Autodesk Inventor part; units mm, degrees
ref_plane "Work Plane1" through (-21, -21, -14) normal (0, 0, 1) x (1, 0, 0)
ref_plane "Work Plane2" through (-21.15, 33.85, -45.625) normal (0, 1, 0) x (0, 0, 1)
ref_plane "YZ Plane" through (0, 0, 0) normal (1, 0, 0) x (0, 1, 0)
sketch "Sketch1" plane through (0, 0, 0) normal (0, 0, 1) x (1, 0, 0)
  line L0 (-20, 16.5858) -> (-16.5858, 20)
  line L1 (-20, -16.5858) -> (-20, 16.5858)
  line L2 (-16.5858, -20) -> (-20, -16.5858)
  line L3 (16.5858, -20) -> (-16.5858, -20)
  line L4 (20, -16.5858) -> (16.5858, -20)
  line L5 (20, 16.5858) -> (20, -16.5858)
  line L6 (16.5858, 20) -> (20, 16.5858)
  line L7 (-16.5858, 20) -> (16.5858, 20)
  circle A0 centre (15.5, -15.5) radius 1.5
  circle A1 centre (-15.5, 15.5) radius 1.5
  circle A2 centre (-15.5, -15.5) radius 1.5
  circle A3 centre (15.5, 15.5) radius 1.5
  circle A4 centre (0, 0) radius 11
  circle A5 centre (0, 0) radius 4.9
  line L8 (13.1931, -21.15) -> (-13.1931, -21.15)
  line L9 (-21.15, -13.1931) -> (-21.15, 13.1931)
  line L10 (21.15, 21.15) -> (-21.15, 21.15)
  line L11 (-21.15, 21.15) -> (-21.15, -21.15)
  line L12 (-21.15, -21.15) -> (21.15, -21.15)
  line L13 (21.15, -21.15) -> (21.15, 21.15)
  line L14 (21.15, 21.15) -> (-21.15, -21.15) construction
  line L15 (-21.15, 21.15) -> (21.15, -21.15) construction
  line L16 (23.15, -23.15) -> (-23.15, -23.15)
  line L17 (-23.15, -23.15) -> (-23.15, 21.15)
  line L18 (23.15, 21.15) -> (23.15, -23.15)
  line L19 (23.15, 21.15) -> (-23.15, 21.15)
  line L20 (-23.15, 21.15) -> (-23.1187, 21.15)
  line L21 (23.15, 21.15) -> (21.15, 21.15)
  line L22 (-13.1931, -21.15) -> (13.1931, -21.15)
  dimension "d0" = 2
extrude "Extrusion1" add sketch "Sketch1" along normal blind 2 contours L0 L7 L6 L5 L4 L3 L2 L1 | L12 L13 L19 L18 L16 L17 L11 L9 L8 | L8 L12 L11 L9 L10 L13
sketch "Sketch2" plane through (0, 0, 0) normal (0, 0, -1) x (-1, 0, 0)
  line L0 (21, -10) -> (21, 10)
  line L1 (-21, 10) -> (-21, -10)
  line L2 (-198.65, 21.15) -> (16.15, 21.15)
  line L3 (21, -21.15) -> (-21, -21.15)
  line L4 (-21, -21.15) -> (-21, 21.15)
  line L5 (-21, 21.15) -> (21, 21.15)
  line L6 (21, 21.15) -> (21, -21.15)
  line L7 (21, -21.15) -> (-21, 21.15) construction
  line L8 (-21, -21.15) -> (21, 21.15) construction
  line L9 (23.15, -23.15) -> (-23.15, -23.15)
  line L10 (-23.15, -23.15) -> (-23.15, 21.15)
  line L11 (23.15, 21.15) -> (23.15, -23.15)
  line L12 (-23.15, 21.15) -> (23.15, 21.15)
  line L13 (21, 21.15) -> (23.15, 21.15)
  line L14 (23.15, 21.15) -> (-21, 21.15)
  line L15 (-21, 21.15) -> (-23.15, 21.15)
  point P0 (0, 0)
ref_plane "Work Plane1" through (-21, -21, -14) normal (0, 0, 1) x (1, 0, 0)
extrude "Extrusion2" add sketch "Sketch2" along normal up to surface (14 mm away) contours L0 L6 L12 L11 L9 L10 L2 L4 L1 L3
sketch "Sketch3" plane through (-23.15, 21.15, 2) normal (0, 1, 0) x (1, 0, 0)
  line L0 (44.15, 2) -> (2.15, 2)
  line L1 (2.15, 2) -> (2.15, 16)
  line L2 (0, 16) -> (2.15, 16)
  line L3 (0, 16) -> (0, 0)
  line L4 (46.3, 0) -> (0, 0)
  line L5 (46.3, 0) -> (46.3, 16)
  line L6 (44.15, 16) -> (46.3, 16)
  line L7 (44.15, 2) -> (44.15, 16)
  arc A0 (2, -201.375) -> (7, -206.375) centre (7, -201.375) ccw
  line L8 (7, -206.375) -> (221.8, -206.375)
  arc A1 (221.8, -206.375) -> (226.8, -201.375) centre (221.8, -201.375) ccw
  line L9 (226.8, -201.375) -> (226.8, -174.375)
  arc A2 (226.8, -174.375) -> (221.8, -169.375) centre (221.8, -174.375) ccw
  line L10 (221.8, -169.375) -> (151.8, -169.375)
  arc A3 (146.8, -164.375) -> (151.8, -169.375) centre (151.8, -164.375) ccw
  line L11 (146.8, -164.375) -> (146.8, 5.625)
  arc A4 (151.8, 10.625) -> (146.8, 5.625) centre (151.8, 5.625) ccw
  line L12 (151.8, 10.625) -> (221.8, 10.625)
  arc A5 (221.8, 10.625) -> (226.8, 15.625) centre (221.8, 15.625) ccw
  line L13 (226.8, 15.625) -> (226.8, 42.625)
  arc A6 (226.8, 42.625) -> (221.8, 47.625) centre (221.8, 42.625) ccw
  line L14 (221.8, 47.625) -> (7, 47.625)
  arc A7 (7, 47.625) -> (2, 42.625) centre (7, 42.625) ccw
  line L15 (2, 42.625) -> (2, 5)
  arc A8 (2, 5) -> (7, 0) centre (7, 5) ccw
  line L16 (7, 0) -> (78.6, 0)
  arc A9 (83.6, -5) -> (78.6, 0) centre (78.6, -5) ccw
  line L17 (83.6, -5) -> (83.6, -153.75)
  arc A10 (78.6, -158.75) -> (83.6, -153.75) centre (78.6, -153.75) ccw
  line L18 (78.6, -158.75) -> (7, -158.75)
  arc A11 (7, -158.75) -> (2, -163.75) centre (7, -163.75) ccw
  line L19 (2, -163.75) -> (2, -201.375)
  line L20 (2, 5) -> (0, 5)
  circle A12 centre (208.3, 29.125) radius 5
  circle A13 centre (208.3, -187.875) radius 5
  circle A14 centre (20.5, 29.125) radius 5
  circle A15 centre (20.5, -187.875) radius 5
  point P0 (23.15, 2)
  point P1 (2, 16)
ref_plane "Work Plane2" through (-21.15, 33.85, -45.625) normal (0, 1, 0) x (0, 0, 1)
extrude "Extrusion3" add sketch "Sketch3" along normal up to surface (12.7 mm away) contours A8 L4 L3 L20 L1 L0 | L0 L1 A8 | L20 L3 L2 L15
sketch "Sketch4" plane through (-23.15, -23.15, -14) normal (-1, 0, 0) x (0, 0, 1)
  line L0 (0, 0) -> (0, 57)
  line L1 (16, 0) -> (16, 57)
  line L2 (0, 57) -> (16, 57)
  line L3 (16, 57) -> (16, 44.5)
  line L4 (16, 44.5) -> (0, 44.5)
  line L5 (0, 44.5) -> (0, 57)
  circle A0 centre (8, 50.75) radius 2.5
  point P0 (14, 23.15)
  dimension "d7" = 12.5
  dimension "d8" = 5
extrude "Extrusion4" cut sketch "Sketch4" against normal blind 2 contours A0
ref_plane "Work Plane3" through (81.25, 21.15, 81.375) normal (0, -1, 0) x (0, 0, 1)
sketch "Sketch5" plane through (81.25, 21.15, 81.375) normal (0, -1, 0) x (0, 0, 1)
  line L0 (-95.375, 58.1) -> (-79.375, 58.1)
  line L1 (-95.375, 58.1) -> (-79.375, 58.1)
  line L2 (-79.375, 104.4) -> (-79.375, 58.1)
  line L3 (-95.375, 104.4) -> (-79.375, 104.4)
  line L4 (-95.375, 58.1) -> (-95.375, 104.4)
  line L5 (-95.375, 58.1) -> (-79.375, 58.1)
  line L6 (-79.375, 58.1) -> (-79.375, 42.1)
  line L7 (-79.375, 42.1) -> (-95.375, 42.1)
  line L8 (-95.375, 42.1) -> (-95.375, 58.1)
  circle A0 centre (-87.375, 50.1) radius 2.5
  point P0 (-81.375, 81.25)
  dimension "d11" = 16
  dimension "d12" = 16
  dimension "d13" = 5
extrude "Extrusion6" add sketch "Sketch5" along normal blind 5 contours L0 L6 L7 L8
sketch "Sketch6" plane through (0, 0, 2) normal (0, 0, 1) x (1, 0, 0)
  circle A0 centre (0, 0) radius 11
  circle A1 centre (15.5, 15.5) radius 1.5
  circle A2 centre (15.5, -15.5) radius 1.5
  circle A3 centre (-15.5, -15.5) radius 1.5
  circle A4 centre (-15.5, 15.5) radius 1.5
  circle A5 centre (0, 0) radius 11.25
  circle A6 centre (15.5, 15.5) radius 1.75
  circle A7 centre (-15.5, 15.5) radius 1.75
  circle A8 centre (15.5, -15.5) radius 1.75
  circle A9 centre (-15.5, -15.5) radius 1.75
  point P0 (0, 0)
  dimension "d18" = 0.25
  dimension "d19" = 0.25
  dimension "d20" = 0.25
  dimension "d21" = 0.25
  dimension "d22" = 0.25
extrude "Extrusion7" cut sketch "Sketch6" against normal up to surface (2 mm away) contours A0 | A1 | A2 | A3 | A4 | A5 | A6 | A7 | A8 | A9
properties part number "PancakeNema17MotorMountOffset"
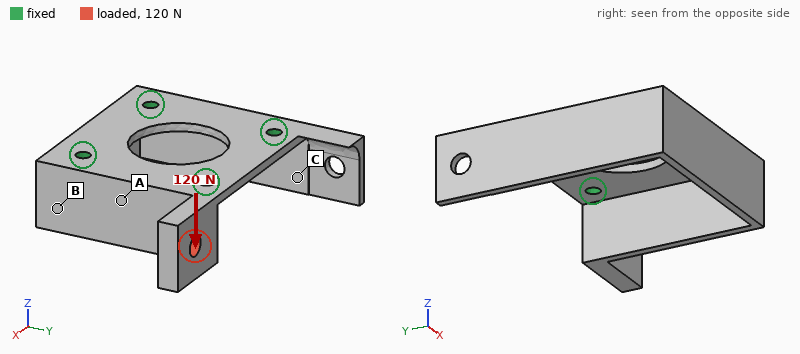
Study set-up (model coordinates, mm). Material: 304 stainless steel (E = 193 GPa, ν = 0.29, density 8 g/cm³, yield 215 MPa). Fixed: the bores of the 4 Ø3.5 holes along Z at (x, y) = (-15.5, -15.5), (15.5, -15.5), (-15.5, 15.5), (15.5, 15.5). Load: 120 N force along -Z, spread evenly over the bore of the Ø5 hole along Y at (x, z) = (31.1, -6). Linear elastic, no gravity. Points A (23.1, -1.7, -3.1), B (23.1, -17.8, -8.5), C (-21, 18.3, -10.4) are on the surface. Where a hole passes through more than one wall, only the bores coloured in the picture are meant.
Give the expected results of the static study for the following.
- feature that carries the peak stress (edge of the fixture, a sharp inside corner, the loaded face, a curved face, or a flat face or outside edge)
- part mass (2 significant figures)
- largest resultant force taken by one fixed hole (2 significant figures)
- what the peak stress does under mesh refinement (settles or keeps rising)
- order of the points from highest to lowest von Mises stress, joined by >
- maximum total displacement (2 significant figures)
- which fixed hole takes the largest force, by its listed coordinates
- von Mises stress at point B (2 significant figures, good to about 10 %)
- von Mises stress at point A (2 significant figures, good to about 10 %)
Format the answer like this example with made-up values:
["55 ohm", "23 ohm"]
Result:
["edge of the fixture", "70 g", "130 N", "keeps rising", "A > B > C", "86 µm", "(15.5, 15.5)", "16 MPa", "28 MPa"]
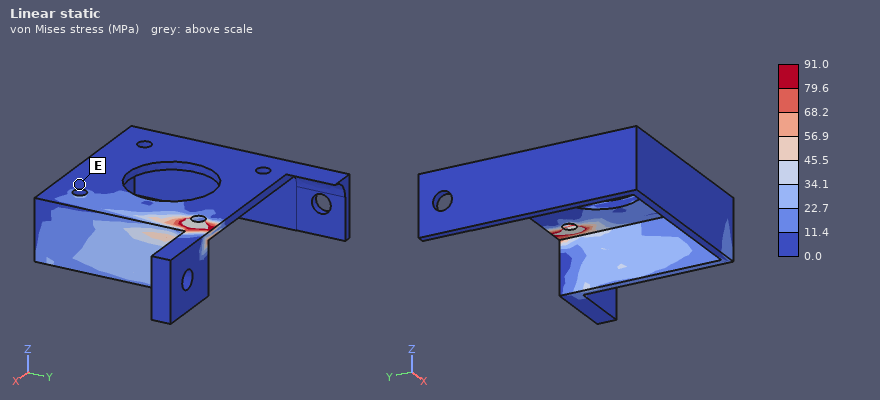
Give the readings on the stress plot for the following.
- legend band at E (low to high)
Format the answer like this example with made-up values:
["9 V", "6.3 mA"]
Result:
["0.0 to 11.4 MPa"]
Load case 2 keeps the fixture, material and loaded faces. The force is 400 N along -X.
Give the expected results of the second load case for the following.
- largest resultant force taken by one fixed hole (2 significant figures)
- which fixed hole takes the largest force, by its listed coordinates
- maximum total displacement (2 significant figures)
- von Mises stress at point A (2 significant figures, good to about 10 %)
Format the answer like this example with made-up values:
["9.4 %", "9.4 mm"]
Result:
["400 N", "(15.5, 15.5)", "0.17 mm", "54 MPa"]
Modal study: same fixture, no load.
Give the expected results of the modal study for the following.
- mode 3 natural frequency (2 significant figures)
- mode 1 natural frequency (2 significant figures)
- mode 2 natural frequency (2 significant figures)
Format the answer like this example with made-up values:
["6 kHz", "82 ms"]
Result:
["5600 Hz", "2000 Hz", "3800 Hz"]
